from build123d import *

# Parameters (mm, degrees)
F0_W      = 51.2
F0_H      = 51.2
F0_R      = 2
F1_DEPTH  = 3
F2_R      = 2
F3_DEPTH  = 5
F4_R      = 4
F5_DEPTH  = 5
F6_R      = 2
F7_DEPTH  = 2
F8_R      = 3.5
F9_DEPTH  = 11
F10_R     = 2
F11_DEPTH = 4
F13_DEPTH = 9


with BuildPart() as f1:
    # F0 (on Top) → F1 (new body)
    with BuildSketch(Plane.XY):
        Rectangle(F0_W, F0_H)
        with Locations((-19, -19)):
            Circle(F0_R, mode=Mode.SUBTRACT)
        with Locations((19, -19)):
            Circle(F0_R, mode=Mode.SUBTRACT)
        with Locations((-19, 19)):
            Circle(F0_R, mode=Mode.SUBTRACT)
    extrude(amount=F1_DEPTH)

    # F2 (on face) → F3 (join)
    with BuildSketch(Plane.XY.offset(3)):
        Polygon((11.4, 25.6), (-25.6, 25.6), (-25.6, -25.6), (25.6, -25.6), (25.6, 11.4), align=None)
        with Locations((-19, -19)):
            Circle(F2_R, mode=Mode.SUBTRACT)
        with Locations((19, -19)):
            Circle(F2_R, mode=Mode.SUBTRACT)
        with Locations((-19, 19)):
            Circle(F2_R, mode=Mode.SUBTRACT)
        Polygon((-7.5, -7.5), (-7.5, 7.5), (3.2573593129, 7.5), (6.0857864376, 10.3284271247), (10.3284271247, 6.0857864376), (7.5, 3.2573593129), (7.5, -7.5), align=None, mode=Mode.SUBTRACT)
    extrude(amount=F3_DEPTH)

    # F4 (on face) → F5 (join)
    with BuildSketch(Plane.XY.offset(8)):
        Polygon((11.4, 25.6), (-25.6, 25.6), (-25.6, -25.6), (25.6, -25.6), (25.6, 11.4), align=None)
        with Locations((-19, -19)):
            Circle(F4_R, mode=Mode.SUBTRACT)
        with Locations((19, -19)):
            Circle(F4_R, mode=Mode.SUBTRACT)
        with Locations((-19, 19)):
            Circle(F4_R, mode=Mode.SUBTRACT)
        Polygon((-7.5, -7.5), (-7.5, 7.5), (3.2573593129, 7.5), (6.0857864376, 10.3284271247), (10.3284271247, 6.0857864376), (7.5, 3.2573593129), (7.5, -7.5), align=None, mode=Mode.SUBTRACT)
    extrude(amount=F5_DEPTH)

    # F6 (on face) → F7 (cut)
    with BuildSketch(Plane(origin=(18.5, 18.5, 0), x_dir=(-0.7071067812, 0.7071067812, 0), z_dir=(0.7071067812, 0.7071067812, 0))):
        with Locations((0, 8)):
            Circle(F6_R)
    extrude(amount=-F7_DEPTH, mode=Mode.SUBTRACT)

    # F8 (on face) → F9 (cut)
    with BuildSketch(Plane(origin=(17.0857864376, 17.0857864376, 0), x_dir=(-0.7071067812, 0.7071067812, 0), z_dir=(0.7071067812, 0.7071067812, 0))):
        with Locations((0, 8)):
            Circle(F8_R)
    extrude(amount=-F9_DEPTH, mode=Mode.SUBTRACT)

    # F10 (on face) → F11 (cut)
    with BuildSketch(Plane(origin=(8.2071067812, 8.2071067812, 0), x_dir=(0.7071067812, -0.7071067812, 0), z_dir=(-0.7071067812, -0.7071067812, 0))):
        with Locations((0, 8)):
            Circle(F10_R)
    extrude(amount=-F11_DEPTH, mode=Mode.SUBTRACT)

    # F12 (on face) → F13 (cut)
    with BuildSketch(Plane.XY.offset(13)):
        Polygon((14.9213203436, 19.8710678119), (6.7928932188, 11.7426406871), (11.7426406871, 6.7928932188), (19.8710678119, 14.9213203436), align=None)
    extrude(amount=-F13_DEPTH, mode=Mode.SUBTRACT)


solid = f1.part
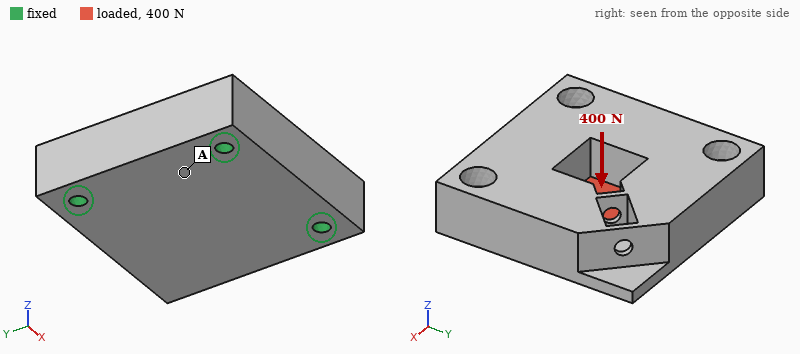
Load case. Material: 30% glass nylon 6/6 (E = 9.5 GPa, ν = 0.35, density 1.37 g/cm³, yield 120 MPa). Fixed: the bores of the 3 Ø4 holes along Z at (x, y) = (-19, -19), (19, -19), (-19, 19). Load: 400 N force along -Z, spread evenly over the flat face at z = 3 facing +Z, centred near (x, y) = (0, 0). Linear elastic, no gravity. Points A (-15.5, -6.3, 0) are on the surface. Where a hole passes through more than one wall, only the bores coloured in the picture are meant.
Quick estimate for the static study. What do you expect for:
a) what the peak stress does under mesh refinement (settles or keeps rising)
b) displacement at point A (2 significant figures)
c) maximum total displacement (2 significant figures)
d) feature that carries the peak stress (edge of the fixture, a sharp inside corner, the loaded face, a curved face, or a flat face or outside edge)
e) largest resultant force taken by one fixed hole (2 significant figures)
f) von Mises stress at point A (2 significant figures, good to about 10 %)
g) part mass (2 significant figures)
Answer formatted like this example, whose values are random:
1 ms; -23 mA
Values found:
keeps rising; 6.5 µm; 39 µm; edge of the fixture; 170 N; 1.8 MPa; 40 g
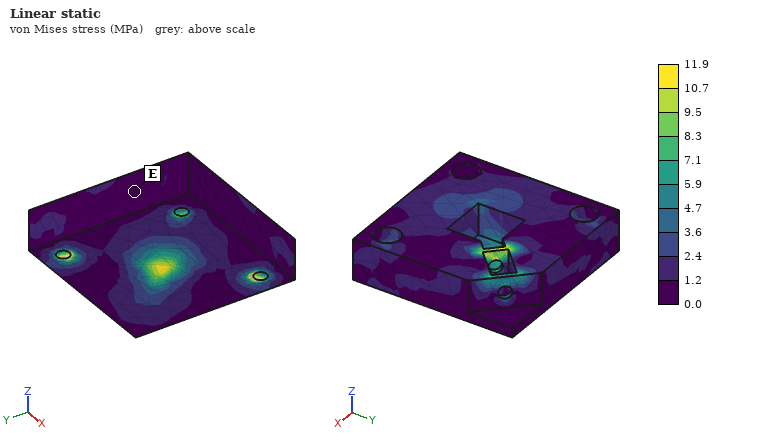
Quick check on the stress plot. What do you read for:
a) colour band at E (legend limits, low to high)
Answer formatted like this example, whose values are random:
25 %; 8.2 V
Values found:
0.0 to 1.2 MPa
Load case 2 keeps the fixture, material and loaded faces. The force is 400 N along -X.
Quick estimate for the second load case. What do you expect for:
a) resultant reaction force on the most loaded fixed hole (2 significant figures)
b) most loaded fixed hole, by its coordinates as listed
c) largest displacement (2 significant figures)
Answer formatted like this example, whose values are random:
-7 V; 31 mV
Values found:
170 N; (-19, 19); 6.9 µm
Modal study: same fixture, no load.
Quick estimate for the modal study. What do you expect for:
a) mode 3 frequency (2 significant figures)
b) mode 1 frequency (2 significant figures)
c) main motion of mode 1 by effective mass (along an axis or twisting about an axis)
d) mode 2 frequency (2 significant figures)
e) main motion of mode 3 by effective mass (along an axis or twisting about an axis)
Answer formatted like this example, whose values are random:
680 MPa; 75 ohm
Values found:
10 kHz; 3900 Hz; along Z; 9600 Hz; along Z
